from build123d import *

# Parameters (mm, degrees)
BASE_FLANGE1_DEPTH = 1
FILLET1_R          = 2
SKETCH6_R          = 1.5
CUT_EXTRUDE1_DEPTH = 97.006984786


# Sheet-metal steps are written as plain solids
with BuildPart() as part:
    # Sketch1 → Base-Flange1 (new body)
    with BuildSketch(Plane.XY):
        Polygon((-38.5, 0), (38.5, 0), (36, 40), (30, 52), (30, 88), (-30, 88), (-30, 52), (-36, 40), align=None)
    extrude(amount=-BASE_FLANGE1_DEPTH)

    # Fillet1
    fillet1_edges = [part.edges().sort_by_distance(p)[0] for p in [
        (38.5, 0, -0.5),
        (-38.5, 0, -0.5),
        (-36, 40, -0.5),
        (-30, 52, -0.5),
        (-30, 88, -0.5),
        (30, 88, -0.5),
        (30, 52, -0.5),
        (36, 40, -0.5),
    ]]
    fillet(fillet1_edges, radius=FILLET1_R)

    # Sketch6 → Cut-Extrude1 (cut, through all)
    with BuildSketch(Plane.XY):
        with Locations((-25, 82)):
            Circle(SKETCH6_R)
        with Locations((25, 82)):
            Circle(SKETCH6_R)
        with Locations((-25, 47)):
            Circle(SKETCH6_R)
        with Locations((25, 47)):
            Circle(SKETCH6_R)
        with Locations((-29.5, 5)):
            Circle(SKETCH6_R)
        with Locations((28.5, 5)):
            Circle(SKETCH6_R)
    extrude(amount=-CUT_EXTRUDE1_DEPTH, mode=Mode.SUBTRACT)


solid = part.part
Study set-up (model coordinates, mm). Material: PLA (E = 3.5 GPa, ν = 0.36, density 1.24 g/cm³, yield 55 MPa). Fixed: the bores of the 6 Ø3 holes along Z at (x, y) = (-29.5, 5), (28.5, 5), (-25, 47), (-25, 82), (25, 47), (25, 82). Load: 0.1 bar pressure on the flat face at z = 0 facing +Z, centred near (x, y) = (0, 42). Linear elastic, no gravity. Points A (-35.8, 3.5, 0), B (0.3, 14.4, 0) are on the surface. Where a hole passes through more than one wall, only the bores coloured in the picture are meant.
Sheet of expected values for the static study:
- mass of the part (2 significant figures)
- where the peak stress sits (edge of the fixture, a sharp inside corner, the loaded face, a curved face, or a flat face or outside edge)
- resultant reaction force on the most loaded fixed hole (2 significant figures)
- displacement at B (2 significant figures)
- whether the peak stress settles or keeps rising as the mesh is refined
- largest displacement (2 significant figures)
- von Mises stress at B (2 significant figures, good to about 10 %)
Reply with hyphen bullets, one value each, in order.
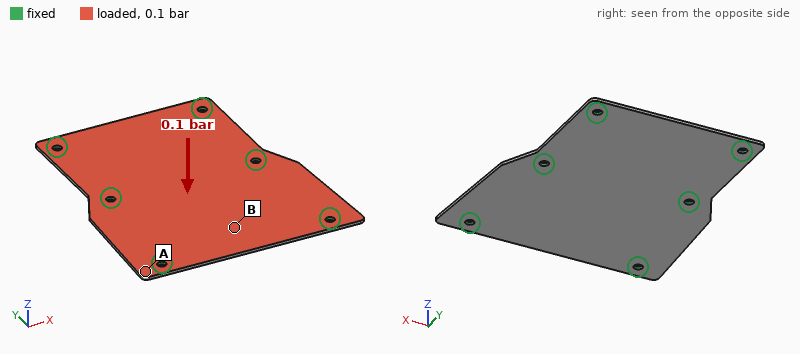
- 7.3 g
- edge of the fixture
- 13 N
- 1.1 mm
- keeps rising
- 1.1 mm
- 7.5 MPa
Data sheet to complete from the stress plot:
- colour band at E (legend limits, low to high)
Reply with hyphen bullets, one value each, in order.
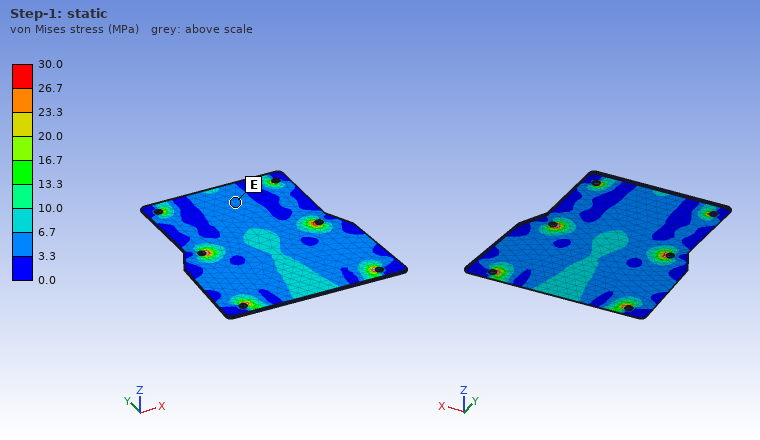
- 3.3 to 6.7 MPa
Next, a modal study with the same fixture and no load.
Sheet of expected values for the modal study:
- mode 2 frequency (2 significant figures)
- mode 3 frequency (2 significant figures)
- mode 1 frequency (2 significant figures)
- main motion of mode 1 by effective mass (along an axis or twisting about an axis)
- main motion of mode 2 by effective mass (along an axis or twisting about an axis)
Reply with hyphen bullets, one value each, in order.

- 650 Hz
- 830 Hz
- 500 Hz
- along Z
- along Z
